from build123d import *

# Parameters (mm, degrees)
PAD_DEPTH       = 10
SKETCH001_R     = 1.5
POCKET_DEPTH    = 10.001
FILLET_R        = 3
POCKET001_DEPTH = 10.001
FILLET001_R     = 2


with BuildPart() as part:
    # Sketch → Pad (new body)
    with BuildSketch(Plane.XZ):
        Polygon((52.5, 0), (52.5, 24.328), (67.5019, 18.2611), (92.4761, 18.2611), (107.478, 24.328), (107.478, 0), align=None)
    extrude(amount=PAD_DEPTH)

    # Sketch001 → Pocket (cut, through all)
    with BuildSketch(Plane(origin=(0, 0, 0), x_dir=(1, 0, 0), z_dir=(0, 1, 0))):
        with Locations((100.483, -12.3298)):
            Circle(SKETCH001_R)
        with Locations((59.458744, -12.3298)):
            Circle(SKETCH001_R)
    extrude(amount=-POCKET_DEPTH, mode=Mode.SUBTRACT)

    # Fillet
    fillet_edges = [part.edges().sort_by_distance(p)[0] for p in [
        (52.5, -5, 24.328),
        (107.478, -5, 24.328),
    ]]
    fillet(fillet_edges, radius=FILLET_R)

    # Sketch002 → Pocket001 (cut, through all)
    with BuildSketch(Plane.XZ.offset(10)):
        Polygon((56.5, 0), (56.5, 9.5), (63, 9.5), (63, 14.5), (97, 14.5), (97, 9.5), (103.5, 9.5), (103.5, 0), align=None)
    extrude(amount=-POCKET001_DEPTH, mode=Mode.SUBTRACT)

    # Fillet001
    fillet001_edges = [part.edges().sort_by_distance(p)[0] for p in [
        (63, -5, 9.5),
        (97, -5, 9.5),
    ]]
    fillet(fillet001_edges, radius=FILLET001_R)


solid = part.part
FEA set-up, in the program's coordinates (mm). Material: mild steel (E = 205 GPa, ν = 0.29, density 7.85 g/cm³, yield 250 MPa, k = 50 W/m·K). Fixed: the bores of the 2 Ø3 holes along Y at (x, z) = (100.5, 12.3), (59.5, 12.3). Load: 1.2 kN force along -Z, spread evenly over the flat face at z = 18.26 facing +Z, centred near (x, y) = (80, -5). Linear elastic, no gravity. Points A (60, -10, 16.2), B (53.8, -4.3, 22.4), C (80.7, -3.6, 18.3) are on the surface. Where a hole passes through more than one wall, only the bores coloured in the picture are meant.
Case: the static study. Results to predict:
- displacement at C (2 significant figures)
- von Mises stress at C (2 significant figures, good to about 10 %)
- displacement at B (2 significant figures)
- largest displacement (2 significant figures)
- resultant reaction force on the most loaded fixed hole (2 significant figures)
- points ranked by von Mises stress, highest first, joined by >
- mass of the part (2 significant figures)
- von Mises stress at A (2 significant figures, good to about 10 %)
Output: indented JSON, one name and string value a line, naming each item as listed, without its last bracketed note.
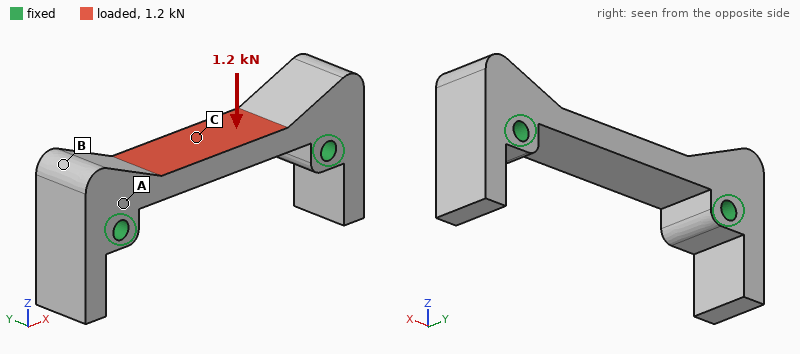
{
  "displacement at C": "22 µm",
  "von Mises stress at C": "100 MPa",
  "displacement at B": "3.7 µm",
  "largest displacement": "23 µm",
  "resultant reaction force on the most loaded fixed hole": "680 N",
  "points ranked by von Mises stress, highest first, joined by >": "C > A > B",
  "mass of the part": "36 g",
  "von Mises stress at A": "36 MPa"
}
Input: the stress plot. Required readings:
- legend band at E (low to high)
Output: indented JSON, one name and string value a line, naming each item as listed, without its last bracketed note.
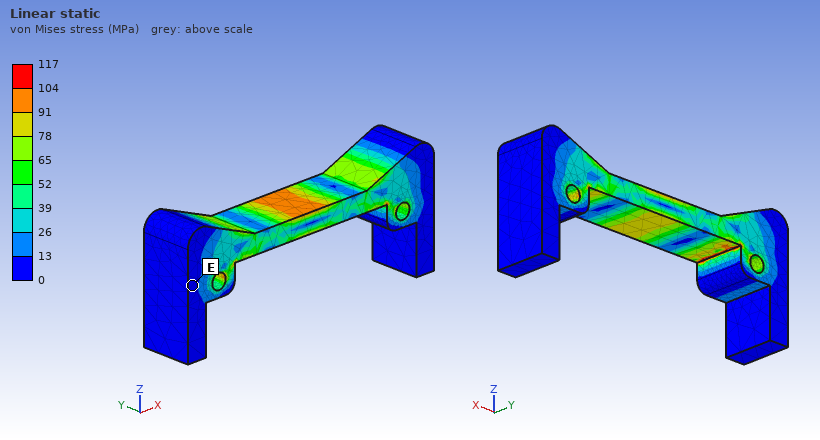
{
  "legend band at E": "0 to 13 MPa"
}
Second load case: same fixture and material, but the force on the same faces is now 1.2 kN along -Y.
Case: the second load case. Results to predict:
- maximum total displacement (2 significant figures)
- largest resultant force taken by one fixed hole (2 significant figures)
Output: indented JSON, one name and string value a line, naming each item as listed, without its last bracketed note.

{
  "maximum total displacement": "11 µm",
  "largest resultant force taken by one fixed hole": "600 N"
}
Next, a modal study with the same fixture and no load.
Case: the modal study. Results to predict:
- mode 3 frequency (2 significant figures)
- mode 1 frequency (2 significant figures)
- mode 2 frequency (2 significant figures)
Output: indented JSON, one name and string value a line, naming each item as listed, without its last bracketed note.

{
  "mode 3 frequency": "21 kHz",
  "mode 1 frequency": "14 kHz",
  "mode 2 frequency": "19 kHz"
}
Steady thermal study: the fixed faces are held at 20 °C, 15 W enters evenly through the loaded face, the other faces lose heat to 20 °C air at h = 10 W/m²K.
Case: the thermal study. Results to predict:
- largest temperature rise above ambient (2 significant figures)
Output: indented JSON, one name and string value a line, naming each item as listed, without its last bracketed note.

{
  "largest temperature rise above ambient": "51 K"
}
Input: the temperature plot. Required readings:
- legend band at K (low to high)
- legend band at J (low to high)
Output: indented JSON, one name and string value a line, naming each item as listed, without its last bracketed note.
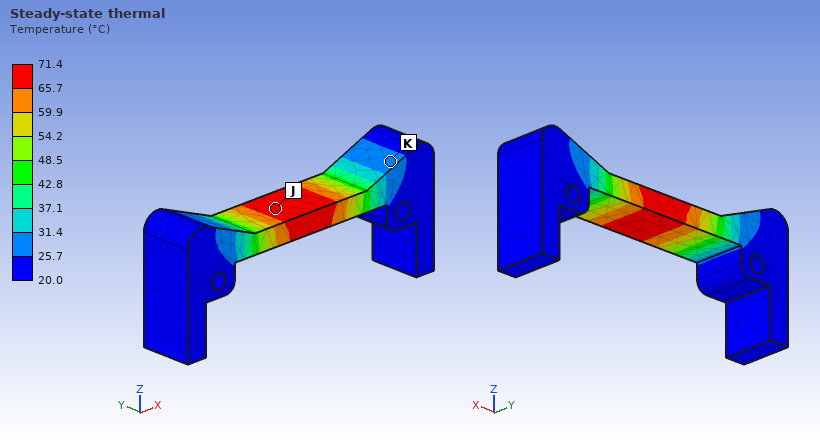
{
  "legend band at K": "25.7 to 31.4 °C",
  "legend band at J": "65.7 to 71.4 °C"
}
